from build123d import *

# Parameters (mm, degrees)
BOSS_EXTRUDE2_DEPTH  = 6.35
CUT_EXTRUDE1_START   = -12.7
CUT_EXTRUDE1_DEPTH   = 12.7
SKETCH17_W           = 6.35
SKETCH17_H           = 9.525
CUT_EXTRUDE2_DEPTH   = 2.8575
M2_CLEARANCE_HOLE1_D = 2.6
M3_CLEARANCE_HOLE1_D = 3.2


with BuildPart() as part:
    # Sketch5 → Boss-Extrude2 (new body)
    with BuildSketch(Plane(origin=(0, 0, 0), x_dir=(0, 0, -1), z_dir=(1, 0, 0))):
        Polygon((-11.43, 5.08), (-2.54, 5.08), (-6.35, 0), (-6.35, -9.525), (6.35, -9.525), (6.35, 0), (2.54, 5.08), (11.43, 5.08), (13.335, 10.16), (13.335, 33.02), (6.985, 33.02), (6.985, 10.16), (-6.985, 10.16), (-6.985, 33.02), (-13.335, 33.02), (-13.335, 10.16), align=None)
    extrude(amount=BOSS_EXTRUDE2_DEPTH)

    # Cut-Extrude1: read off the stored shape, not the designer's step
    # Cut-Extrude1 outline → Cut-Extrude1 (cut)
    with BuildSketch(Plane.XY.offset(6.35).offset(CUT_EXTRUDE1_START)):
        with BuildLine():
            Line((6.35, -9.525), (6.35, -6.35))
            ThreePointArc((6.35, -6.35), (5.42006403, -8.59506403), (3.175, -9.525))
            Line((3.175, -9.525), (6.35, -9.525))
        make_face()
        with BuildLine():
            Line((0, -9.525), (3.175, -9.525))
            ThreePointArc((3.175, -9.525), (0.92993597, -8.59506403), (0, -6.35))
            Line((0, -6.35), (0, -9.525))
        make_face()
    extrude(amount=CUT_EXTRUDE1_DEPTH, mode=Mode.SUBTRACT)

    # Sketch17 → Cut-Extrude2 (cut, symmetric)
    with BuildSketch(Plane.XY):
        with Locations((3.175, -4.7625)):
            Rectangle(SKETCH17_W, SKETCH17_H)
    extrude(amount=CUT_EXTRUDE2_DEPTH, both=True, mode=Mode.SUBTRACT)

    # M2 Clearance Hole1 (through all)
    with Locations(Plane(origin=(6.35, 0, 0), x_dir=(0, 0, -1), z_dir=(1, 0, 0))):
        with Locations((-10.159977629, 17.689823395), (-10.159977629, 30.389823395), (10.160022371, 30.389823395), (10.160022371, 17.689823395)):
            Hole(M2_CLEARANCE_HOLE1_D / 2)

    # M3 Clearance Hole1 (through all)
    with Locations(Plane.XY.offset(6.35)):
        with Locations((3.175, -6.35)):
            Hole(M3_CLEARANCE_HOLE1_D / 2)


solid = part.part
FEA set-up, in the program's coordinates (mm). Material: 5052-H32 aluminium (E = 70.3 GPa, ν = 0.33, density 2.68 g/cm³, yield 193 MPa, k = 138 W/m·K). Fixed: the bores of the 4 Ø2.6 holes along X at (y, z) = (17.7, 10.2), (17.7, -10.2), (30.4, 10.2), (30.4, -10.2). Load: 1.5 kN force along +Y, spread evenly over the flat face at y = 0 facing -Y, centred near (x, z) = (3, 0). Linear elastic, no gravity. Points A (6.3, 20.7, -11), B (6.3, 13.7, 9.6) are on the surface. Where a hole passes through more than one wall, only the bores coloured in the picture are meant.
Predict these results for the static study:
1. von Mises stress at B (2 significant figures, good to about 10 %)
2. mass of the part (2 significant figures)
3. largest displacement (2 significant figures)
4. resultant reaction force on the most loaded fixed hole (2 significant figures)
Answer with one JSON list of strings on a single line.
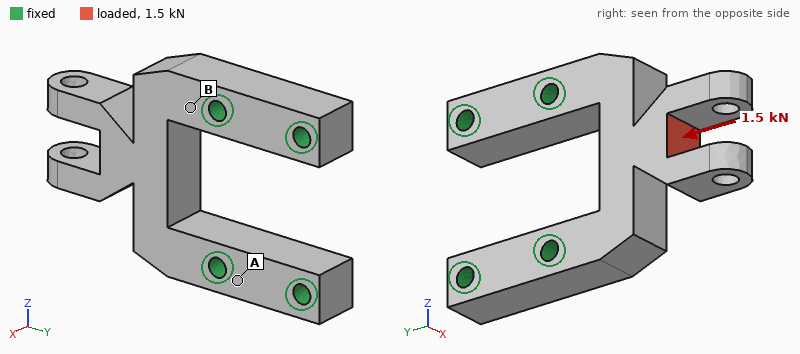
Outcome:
["38 MPa", "8.4 g", "20 µm", "830 N"]
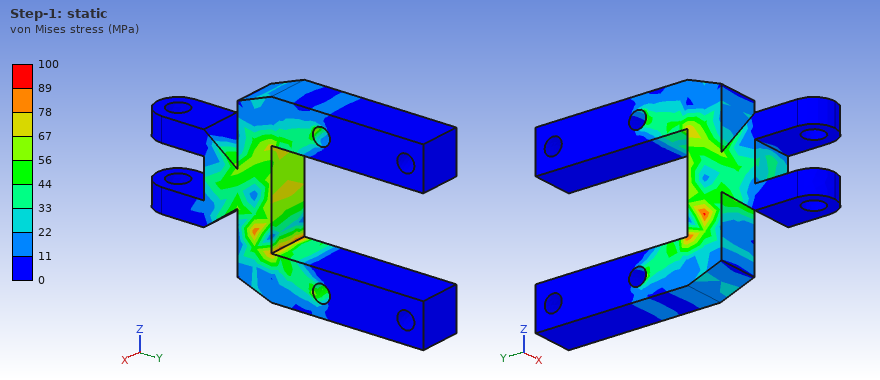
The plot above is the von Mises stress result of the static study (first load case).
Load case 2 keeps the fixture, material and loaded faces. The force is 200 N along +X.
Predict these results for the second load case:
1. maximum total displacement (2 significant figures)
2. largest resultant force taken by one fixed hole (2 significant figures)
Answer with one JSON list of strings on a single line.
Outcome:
["61 µm", "110 N"]
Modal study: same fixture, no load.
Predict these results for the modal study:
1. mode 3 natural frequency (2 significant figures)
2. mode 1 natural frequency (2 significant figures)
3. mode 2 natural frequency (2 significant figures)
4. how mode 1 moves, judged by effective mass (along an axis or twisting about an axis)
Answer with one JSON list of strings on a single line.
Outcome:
["19 kHz", "7700 Hz", "13 kHz", "along X"]
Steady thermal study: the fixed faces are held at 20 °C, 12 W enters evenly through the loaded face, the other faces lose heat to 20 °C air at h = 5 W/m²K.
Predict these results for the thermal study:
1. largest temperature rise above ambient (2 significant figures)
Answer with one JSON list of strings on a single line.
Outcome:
["32 K"]
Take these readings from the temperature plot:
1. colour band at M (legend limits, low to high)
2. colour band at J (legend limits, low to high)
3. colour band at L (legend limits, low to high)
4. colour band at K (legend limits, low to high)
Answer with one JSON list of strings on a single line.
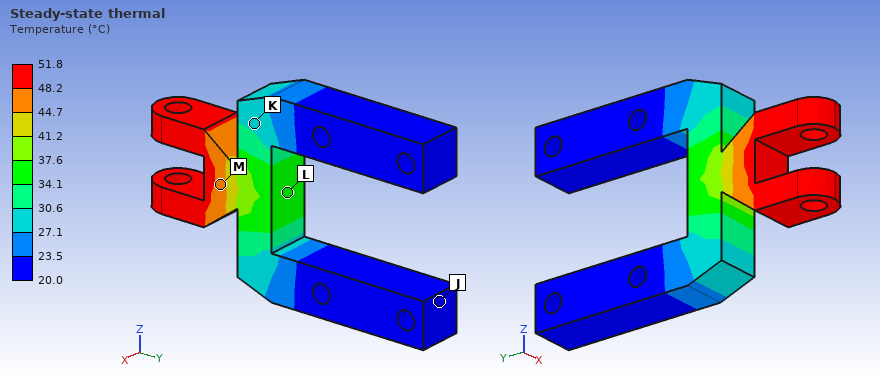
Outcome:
["44.7 to 48.2 °C", "20.0 to 23.5 °C", "34.1 to 37.6 °C", "27.1 to 30.6 °C"]
